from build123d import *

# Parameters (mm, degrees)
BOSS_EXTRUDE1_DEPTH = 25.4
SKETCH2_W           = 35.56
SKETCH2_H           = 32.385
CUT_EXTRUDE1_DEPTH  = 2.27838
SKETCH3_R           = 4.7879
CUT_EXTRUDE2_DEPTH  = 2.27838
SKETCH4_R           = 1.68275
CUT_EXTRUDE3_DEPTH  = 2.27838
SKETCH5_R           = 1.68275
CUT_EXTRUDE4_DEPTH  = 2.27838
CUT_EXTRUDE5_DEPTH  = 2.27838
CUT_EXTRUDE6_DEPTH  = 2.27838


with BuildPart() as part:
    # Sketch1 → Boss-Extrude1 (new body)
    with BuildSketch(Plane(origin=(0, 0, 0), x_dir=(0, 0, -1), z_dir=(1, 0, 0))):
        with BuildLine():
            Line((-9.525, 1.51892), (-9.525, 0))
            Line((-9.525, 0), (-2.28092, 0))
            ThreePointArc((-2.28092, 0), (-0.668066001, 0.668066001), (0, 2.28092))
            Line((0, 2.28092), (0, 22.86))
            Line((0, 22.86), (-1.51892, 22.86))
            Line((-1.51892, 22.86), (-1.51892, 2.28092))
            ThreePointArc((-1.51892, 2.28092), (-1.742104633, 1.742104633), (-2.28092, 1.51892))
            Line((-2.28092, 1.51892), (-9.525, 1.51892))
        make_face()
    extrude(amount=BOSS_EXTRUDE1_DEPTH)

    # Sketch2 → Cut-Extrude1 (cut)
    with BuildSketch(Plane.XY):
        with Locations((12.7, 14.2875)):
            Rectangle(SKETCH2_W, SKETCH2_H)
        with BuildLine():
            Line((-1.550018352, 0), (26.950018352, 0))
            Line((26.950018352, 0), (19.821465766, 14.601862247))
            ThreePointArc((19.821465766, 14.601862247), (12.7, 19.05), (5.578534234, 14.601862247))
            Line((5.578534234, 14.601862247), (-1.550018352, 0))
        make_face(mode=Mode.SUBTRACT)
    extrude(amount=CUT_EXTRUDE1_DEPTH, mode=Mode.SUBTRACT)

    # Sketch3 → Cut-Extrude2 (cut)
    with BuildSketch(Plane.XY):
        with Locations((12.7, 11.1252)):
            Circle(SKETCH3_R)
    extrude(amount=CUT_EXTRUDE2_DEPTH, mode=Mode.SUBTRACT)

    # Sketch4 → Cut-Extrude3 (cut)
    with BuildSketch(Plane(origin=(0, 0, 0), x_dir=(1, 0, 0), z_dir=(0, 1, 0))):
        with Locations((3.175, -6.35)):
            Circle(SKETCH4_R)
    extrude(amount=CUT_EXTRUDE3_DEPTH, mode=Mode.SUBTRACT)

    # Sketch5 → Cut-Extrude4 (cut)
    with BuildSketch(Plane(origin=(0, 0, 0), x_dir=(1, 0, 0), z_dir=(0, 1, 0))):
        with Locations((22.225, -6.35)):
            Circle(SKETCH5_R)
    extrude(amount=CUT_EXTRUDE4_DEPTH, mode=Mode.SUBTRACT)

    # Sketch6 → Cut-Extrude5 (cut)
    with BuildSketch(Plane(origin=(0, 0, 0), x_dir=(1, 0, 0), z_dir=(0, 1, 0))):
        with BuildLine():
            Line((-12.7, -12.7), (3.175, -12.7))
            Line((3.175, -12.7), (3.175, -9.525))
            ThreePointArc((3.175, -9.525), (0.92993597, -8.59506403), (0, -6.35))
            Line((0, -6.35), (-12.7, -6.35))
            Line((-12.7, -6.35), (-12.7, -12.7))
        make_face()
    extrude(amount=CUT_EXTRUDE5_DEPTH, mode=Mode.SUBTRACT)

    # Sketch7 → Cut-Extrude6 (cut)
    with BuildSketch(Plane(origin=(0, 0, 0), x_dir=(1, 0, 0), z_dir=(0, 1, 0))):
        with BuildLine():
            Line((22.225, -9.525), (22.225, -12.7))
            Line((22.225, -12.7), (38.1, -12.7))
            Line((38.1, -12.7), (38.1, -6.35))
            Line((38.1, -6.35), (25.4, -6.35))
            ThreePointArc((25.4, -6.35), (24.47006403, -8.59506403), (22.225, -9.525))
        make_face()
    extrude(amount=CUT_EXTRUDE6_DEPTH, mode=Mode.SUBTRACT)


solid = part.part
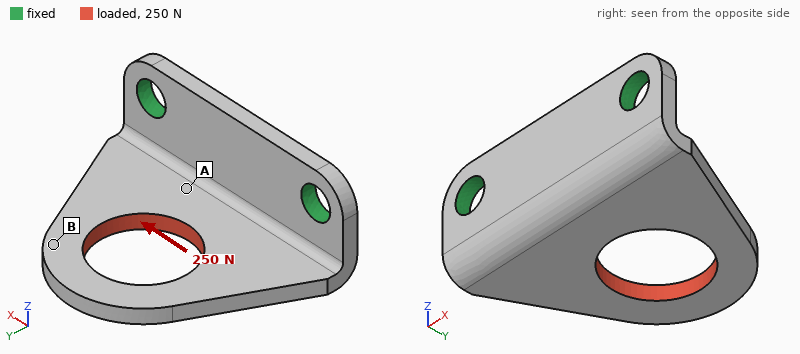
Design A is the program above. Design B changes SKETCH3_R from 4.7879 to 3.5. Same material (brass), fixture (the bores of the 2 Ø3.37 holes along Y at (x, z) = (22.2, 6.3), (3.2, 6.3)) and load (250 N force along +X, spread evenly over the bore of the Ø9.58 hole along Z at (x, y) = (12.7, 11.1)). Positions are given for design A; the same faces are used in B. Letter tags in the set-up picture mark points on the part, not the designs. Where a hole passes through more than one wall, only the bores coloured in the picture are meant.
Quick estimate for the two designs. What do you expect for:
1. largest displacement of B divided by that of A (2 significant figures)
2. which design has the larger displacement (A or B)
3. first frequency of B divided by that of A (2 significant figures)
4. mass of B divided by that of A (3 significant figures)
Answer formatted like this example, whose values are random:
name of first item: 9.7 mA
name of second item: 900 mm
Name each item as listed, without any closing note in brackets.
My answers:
largest displacement of B divided by that of A: 0.88
which design has the larger displacement: A
first frequency of B divided by that of A: 0.95
mass of B divided by that of A: 1.08
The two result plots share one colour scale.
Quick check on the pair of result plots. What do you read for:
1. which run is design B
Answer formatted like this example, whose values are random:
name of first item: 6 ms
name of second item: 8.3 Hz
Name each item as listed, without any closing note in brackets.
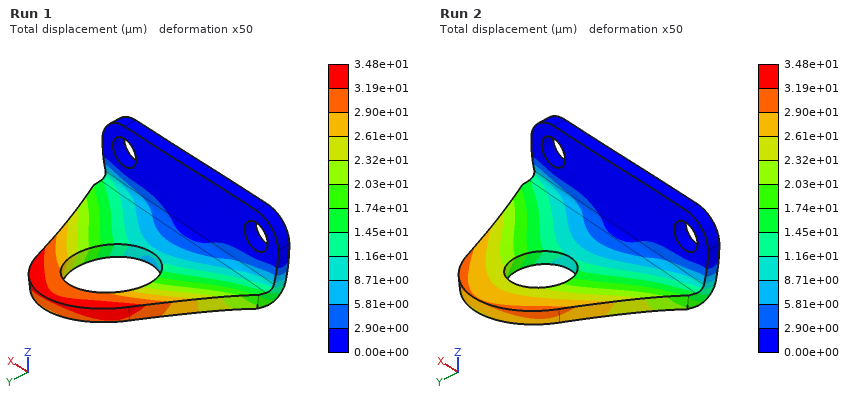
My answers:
which run is design B: Run 2
